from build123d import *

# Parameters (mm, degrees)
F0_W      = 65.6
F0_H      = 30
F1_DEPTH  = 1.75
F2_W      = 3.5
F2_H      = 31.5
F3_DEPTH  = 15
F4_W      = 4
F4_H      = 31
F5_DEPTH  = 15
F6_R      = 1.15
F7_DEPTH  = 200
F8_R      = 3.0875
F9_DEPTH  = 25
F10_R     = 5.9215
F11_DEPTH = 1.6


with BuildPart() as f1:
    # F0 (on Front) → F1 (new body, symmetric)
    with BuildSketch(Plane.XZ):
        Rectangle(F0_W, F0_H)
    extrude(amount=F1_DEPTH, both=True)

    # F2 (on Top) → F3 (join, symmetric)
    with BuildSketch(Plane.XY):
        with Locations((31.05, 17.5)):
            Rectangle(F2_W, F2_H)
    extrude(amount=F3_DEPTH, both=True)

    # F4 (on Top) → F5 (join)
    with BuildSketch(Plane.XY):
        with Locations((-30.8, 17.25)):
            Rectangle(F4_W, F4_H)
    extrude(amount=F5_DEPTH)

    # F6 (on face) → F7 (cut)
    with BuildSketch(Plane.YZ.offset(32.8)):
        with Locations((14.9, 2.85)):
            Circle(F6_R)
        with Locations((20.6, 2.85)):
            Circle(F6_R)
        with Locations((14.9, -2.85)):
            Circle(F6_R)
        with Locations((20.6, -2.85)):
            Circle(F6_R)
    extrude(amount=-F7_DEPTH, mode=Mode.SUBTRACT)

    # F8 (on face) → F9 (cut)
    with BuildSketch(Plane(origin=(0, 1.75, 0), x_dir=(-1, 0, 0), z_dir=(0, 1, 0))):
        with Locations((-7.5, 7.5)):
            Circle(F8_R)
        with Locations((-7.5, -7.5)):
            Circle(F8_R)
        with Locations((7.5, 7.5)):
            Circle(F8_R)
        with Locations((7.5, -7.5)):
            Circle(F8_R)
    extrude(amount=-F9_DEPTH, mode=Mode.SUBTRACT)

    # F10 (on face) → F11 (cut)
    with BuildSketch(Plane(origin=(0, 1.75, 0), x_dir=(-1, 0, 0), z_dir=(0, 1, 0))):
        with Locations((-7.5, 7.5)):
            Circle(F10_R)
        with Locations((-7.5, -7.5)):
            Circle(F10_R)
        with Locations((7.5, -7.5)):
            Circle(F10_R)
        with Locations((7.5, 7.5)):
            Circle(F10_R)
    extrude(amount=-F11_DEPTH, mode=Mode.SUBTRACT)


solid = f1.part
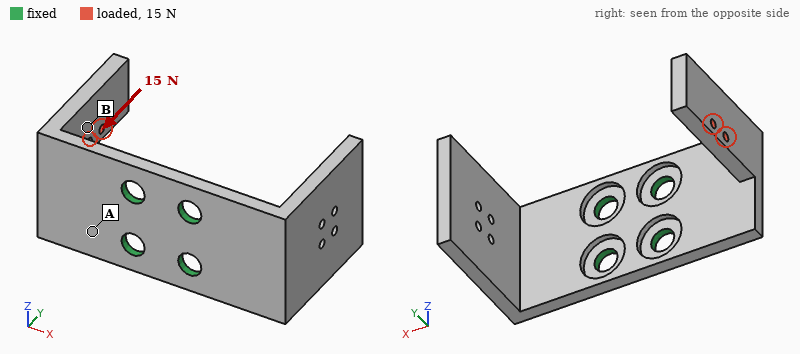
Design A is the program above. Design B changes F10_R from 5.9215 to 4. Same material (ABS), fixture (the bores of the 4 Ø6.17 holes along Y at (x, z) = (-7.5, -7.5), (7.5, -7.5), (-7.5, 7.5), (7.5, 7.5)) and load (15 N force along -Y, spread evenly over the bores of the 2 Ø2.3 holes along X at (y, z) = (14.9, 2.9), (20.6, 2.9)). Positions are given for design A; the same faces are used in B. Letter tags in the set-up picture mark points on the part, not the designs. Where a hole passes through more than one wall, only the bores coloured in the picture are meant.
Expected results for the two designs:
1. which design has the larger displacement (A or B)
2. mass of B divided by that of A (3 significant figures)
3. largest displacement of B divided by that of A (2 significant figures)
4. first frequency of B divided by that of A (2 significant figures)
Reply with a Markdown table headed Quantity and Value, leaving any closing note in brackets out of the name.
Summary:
| Quantity | Value |
|---|---|
| which design has the larger displacement | A |
| mass of B divided by that of A | 1.03 |
| largest displacement of B divided by that of A | 0.80 |
| first frequency of B divided by that of A | 1.1 |
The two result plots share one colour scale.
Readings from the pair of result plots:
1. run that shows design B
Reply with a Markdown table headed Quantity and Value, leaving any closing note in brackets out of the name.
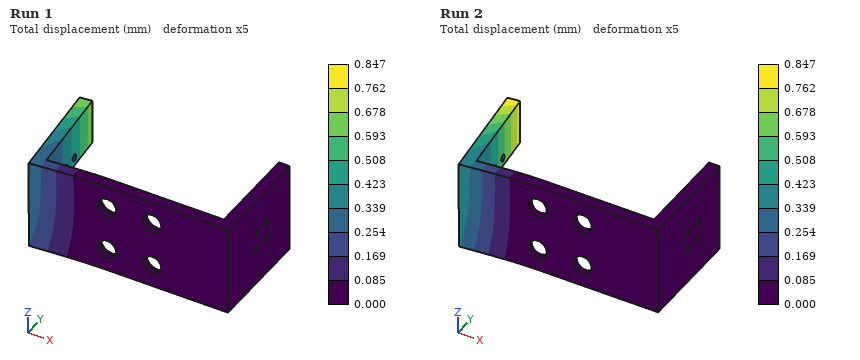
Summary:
| Quantity | Value |
|---|---|
| run that shows design B | Run 1 |
